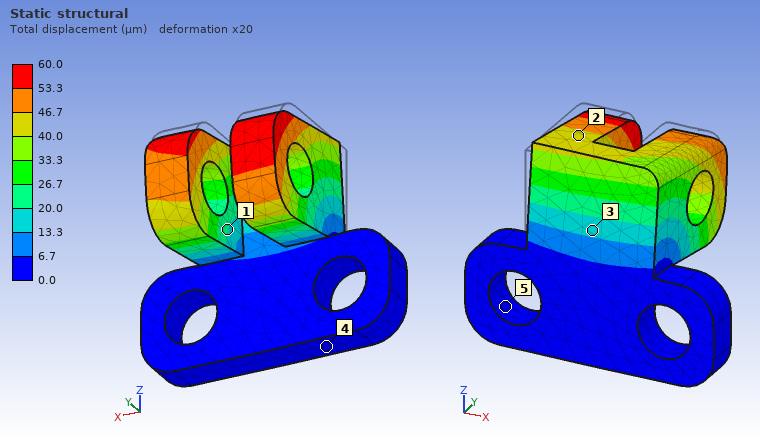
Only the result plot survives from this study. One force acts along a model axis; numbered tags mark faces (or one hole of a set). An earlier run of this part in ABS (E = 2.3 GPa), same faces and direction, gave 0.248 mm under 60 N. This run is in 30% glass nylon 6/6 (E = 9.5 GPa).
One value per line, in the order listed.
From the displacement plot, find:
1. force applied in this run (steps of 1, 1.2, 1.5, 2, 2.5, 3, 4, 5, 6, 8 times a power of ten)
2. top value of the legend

60 N
60.0 µm
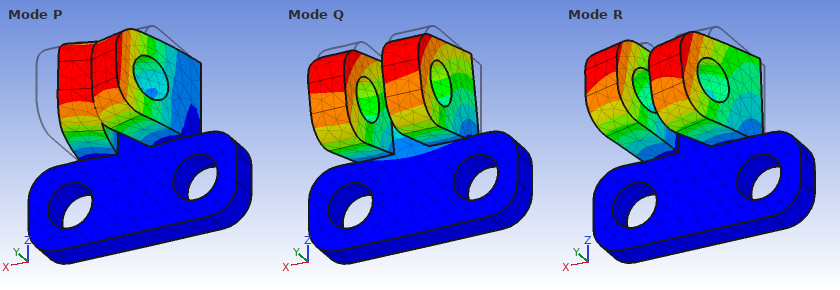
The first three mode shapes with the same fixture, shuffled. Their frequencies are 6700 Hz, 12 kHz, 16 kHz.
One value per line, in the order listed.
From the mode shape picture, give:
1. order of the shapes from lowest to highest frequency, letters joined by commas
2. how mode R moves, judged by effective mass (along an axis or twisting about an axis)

Q, R, P
along X
